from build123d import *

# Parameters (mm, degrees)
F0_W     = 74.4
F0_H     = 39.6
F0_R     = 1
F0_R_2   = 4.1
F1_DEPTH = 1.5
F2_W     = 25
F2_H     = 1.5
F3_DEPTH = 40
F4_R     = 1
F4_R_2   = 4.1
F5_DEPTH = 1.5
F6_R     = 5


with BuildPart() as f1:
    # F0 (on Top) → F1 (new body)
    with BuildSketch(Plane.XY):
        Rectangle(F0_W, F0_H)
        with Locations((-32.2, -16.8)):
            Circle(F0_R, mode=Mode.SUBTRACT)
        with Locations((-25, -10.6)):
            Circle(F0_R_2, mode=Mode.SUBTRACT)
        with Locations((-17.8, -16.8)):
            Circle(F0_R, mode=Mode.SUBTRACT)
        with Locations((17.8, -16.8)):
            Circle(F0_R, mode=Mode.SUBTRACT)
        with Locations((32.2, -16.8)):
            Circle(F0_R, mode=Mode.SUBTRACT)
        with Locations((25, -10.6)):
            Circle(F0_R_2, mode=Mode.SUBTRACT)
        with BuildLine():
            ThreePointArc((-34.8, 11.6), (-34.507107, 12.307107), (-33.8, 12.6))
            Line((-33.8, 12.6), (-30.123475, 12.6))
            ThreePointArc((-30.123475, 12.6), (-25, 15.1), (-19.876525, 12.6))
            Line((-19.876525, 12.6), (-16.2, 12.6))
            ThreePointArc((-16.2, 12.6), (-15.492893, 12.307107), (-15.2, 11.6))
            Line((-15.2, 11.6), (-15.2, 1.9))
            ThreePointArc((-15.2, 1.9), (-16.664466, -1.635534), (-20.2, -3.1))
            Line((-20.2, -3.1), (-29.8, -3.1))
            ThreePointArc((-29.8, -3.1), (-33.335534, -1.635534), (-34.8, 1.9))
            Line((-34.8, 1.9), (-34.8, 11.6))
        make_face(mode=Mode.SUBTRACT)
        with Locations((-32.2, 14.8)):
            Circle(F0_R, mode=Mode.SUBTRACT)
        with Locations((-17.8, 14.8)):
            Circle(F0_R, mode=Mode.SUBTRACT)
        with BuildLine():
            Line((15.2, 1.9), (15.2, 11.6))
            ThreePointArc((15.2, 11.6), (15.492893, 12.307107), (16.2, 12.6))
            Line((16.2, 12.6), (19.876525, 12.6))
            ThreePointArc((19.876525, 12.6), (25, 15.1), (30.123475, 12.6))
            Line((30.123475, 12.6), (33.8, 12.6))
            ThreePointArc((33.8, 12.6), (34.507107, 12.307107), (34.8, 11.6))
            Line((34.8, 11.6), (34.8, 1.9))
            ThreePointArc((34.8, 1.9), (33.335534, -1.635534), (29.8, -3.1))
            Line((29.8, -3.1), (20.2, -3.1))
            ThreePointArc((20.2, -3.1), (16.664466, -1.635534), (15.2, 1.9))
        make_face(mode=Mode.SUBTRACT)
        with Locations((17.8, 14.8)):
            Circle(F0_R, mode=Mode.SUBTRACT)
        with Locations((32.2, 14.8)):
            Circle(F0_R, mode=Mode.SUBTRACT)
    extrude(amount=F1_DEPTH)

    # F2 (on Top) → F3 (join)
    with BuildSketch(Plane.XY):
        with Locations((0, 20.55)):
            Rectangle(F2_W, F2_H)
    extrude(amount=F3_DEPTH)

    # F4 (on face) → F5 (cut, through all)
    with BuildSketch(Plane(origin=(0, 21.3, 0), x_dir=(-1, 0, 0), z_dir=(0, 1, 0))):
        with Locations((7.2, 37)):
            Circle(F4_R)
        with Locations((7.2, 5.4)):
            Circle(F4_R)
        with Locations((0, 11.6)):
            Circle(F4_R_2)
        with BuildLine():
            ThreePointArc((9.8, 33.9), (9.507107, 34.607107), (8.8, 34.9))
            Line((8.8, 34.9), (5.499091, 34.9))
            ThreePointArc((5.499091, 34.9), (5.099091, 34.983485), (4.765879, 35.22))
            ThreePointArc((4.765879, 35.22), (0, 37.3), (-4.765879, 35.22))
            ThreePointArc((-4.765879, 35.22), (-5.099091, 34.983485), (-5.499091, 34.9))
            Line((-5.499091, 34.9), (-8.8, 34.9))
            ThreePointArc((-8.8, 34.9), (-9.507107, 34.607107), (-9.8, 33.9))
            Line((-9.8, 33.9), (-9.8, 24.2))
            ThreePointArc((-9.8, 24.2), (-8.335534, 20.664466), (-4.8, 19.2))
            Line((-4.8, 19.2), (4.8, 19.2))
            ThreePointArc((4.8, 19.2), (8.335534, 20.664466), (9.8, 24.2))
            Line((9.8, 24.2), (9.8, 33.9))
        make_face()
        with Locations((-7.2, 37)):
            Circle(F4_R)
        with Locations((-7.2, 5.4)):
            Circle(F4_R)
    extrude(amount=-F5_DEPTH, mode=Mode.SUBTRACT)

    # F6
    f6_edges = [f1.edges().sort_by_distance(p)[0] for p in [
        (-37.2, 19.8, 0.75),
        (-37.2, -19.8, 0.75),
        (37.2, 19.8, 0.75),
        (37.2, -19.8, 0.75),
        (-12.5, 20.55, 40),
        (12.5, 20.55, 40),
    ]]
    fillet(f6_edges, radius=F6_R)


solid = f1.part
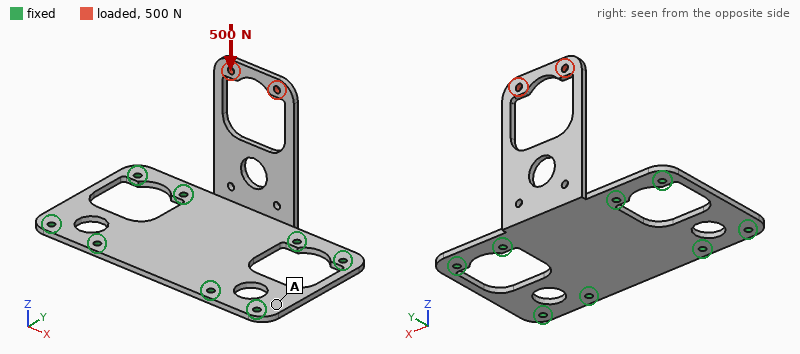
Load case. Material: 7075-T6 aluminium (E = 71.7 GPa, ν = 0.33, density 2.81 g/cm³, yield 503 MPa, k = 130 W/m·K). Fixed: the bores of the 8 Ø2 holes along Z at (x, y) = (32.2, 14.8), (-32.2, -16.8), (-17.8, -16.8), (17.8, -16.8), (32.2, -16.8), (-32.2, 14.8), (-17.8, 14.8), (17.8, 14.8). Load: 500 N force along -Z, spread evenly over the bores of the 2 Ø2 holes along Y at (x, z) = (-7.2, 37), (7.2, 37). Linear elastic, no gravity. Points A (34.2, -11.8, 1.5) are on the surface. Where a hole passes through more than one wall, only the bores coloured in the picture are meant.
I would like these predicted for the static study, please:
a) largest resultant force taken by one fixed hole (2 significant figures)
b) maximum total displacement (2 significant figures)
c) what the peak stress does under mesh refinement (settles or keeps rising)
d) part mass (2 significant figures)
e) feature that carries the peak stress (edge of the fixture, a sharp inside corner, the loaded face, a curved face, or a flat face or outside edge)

290 N
0.96 mm
keeps rising
12 g
edge of the fixture
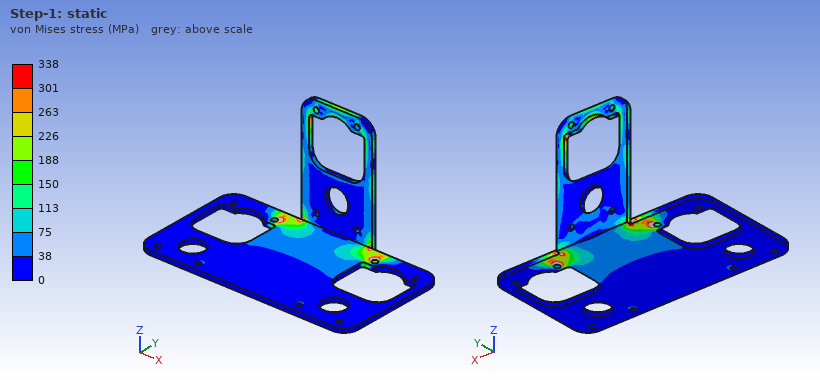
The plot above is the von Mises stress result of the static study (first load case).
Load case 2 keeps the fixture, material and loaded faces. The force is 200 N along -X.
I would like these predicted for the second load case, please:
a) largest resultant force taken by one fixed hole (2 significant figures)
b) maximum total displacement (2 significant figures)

280 N
0.73 mm
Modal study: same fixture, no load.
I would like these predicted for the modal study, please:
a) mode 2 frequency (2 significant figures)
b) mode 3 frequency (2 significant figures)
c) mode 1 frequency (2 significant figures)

2400 Hz
3200 Hz
790 Hz
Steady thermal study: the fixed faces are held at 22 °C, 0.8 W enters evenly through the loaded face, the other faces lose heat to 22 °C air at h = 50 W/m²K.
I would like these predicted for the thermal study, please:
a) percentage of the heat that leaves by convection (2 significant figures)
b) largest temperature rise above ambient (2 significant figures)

53 %
14 K
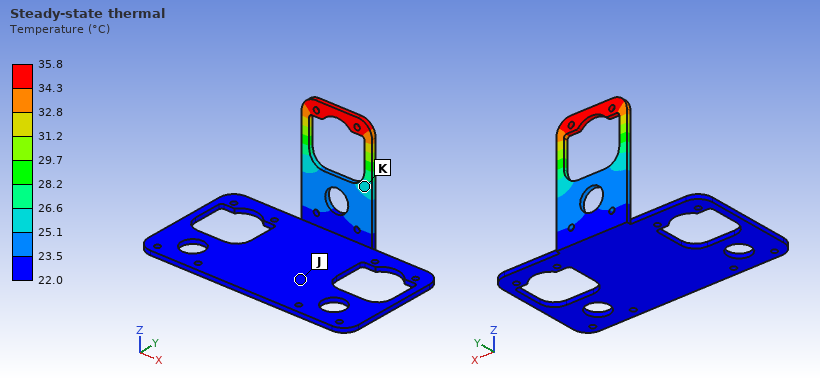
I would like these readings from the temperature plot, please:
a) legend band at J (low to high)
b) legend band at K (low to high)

22.0 to 23.5 °C
25.1 to 26.6 °C
